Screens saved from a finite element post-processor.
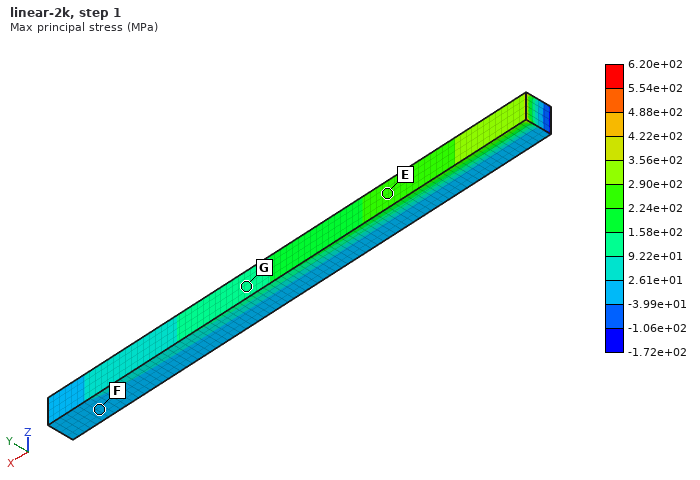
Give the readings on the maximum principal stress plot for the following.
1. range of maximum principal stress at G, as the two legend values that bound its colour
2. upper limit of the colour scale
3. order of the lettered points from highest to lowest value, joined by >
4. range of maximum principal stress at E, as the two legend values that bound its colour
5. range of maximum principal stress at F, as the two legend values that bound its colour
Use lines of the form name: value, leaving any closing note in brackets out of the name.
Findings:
range of maximum principal stress at G, as the two legend values that bound its colour: 9.22e+01 to 1.58e+02 MPa
upper limit of the colour scale: 6.20e+02 MPa
order of the lettered points from highest to lowest value, joined by >: E > G > F
range of maximum principal stress at E, as the two legend values that bound its colour: 2.24e+02 to 2.90e+02 MPa
range of maximum principal stress at F, as the two legend values that bound its colour: -3.99e+01 to 2.61e+01 MPa
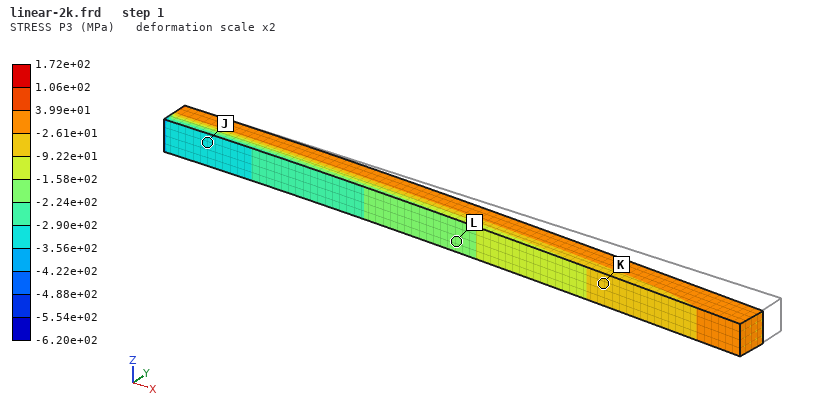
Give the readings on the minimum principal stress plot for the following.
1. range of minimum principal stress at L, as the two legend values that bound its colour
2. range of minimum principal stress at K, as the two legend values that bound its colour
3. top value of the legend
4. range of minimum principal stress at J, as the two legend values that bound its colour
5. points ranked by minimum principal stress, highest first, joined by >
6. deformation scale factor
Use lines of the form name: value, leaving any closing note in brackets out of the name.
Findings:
range of minimum principal stress at L, as the two legend values that bound its colour: -2.24e+02 to -1.58e+02 MPa
range of minimum principal stress at K, as the two legend values that bound its colour: -9.22e+01 to -2.61e+01 MPa
top value of the legend: 1.72e+02 MPa
range of minimum principal stress at J, as the two legend values that bound its colour: -3.56e+02 to -2.90e+02 MPa
points ranked by minimum principal stress, highest first, joined by >: K > L > J
deformation scale factor: 2
